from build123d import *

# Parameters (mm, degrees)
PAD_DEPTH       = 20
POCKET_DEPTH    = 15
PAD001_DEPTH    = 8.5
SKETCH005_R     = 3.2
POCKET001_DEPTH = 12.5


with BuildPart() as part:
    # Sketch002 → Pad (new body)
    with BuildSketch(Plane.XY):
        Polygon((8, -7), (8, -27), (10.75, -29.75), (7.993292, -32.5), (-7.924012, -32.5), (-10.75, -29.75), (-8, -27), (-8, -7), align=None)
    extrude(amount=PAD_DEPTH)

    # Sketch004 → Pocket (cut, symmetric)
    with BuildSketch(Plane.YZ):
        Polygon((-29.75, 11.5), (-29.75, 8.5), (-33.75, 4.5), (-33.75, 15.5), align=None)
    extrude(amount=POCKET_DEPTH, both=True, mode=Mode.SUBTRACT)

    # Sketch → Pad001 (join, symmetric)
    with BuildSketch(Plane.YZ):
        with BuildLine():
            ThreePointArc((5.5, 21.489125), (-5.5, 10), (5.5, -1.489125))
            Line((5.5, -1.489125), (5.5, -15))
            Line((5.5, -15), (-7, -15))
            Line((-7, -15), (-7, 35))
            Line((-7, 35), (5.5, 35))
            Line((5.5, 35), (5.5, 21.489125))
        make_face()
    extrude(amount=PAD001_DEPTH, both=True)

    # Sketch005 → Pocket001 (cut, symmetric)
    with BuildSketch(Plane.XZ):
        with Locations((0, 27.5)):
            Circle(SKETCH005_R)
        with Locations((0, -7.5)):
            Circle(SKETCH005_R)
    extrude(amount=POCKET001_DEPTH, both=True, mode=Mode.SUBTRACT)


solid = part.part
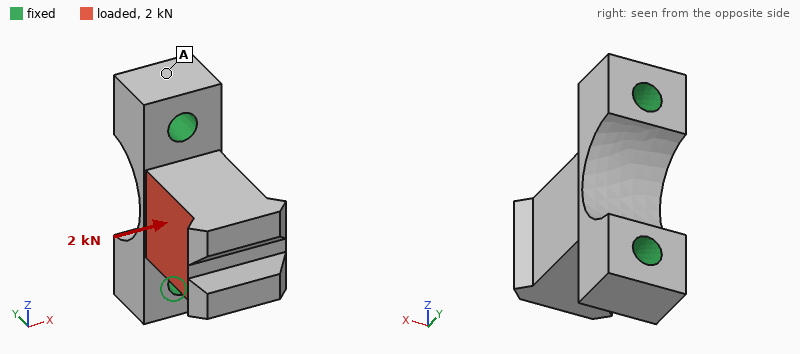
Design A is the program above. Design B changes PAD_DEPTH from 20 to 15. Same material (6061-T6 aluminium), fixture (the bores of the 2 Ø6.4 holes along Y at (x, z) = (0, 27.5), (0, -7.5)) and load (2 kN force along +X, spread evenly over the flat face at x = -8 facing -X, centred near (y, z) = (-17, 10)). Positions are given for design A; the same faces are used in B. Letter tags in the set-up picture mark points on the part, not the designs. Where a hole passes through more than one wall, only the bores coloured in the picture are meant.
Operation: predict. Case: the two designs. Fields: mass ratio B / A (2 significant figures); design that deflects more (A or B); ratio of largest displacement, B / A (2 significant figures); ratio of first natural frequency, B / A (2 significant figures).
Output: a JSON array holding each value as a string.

["0.86", "B", "1.4", "0.98"]
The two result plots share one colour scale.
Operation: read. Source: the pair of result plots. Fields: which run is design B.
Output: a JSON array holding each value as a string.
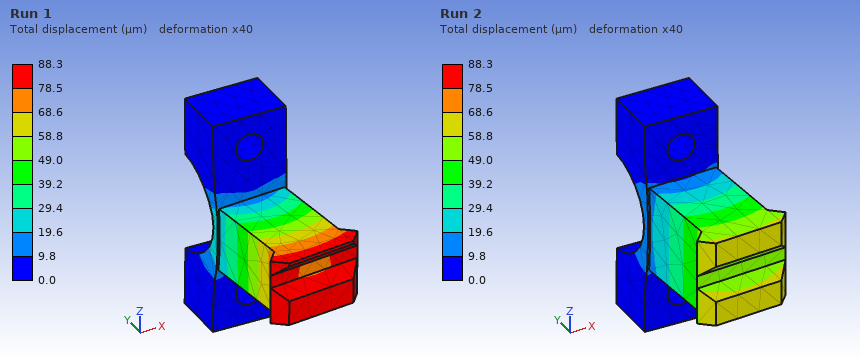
["Run 1"]
